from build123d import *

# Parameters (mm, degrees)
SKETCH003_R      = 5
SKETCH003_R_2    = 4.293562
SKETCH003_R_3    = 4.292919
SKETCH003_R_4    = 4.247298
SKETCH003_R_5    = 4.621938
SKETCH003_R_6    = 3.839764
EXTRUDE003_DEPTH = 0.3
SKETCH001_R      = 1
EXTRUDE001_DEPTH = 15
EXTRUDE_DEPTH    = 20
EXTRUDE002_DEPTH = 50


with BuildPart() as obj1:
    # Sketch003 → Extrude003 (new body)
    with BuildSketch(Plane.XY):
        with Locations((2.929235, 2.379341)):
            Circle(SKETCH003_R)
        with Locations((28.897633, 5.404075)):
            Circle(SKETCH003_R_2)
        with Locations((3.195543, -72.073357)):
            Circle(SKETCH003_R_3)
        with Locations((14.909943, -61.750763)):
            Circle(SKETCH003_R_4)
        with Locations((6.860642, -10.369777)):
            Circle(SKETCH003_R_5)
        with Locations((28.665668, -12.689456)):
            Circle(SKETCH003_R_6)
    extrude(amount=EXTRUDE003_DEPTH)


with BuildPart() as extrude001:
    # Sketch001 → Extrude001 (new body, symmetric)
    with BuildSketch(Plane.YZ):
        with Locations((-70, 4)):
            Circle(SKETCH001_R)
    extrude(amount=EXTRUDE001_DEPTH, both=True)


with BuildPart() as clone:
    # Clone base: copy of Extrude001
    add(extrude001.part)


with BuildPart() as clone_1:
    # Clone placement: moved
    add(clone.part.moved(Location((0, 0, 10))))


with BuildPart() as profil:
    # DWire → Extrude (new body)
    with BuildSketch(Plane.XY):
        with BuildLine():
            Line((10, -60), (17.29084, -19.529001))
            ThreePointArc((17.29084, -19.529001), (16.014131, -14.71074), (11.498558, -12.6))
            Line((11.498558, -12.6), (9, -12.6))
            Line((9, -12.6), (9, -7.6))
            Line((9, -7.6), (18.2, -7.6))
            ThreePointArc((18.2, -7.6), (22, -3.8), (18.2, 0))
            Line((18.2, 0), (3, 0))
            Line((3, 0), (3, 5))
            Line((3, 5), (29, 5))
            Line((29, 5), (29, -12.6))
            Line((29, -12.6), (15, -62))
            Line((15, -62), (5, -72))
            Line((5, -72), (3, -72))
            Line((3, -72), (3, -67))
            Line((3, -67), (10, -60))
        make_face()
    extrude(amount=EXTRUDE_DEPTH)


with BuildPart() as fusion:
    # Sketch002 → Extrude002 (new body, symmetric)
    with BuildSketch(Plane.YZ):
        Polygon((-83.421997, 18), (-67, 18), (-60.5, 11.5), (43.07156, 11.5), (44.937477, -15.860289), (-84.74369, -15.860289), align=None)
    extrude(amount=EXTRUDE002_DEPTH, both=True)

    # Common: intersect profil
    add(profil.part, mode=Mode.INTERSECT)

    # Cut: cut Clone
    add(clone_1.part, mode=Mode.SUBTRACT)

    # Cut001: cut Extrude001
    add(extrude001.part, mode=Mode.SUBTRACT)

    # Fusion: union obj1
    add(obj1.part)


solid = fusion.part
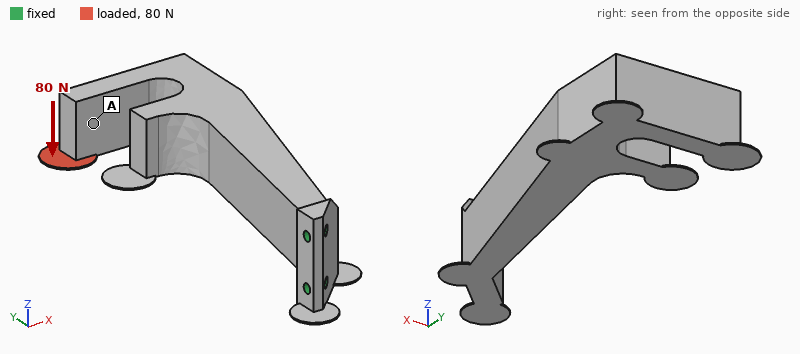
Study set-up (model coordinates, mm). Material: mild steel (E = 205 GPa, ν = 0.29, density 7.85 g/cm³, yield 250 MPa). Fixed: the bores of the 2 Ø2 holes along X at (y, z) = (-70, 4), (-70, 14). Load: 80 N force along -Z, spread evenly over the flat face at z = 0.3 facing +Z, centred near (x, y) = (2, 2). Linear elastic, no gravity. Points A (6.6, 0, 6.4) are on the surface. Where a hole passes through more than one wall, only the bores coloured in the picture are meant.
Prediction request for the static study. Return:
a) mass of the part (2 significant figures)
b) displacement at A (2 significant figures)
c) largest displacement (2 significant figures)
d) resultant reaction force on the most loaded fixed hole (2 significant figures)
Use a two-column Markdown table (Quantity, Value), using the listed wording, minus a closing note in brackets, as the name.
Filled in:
| Quantity | Value |
|---|---|
| mass of the part | 70 g |
| displacement at A | 0.12 mm |
| largest displacement | 0.26 mm |
| resultant reaction force on the most loaded fixed hole | 560 N |
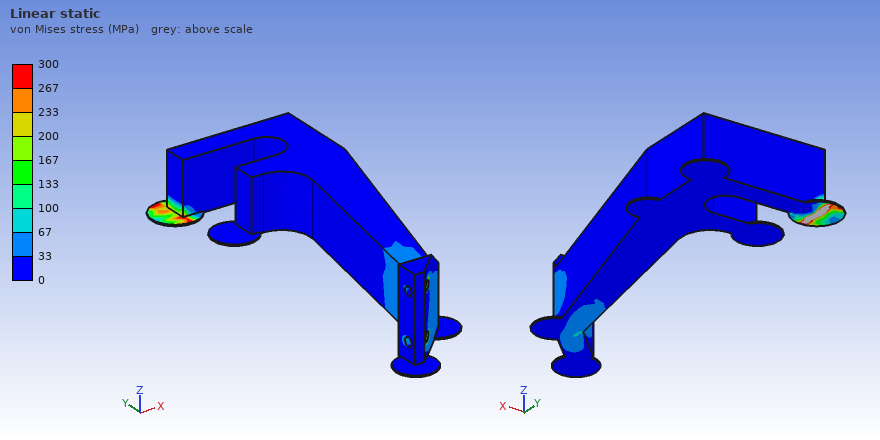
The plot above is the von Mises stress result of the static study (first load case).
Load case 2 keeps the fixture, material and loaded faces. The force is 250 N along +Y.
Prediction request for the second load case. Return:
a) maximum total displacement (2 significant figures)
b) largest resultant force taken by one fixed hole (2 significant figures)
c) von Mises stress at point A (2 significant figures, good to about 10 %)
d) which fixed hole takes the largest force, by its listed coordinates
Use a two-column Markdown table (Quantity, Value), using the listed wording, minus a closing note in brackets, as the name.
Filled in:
| Quantity | Value |
|---|---|
| maximum total displacement | 0.22 mm |
| largest resultant force taken by one fixed hole | 320 N |
| von Mises stress at point A | 38 MPa |
| which fixed hole takes the largest force, by its listed coordinates | (-70, 4) |
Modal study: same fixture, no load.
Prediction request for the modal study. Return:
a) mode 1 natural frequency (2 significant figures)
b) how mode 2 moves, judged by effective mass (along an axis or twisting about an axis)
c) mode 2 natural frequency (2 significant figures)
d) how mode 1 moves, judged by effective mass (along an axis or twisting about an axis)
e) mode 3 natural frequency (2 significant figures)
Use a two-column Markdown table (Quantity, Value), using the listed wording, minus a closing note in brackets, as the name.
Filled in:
| Quantity | Value |
|---|---|
| mode 1 natural frequency | 480 Hz |
| how mode 2 moves, judged by effective mass | along Z |
| mode 2 natural frequency | 930 Hz |
| how mode 1 moves, judged by effective mass | along X |
| mode 3 natural frequency | 3500 Hz |
